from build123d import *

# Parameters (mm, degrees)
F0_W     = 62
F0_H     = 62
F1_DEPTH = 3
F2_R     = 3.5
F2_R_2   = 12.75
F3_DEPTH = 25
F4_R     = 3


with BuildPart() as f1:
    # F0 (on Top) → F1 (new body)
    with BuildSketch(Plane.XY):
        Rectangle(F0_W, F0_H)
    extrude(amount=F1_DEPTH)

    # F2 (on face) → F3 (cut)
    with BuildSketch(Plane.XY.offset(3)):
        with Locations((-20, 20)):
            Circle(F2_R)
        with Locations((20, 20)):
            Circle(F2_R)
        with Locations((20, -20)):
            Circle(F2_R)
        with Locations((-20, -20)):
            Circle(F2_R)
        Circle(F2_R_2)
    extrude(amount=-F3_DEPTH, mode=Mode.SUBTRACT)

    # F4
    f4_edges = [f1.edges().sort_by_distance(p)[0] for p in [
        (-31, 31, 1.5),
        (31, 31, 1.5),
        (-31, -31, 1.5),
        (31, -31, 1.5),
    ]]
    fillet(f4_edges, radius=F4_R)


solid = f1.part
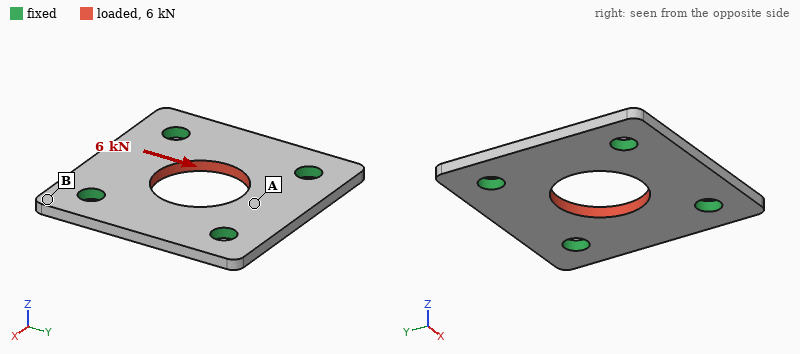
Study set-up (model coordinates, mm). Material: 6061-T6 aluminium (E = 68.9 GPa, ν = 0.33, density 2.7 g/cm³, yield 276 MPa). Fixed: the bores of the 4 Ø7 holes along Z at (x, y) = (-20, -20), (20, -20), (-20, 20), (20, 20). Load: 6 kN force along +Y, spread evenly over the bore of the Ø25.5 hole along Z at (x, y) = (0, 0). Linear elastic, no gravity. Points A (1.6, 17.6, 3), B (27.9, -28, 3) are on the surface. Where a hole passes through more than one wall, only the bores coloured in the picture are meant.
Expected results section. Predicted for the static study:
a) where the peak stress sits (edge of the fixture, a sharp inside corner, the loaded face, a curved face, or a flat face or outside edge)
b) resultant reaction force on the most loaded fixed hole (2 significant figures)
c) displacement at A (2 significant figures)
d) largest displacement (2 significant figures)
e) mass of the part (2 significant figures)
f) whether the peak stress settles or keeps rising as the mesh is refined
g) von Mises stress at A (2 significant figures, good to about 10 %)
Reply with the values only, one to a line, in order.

edge of the fixture
1.6 kN
11 µm
13 µm
26 g
keeps rising
18 MPa
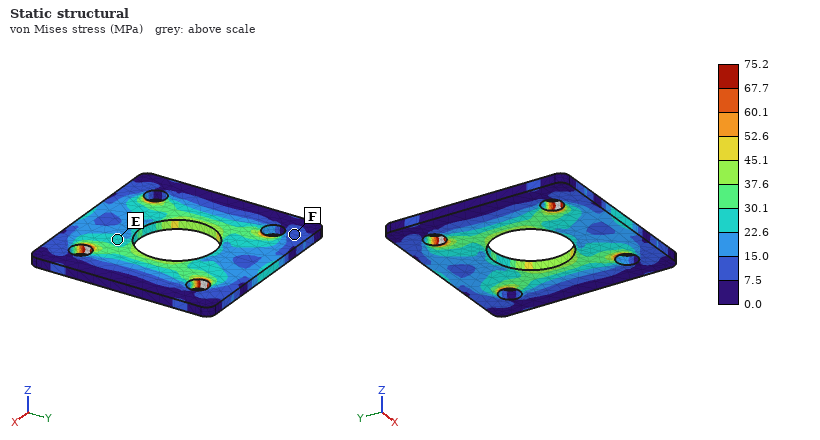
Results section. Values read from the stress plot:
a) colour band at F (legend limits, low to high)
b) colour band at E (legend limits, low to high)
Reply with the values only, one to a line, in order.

7.5 to 15.0 MPa
22.6 to 30.1 MPa
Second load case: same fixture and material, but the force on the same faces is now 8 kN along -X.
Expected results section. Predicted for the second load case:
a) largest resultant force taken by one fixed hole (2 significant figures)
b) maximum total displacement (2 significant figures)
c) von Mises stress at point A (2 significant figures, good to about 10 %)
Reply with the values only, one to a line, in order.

2.1 kN
17 µm
36 MPa
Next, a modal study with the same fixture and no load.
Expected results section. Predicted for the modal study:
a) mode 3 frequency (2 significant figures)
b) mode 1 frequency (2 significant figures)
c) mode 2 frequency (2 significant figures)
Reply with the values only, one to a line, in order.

11 kHz
11 kHz
11 kHz
